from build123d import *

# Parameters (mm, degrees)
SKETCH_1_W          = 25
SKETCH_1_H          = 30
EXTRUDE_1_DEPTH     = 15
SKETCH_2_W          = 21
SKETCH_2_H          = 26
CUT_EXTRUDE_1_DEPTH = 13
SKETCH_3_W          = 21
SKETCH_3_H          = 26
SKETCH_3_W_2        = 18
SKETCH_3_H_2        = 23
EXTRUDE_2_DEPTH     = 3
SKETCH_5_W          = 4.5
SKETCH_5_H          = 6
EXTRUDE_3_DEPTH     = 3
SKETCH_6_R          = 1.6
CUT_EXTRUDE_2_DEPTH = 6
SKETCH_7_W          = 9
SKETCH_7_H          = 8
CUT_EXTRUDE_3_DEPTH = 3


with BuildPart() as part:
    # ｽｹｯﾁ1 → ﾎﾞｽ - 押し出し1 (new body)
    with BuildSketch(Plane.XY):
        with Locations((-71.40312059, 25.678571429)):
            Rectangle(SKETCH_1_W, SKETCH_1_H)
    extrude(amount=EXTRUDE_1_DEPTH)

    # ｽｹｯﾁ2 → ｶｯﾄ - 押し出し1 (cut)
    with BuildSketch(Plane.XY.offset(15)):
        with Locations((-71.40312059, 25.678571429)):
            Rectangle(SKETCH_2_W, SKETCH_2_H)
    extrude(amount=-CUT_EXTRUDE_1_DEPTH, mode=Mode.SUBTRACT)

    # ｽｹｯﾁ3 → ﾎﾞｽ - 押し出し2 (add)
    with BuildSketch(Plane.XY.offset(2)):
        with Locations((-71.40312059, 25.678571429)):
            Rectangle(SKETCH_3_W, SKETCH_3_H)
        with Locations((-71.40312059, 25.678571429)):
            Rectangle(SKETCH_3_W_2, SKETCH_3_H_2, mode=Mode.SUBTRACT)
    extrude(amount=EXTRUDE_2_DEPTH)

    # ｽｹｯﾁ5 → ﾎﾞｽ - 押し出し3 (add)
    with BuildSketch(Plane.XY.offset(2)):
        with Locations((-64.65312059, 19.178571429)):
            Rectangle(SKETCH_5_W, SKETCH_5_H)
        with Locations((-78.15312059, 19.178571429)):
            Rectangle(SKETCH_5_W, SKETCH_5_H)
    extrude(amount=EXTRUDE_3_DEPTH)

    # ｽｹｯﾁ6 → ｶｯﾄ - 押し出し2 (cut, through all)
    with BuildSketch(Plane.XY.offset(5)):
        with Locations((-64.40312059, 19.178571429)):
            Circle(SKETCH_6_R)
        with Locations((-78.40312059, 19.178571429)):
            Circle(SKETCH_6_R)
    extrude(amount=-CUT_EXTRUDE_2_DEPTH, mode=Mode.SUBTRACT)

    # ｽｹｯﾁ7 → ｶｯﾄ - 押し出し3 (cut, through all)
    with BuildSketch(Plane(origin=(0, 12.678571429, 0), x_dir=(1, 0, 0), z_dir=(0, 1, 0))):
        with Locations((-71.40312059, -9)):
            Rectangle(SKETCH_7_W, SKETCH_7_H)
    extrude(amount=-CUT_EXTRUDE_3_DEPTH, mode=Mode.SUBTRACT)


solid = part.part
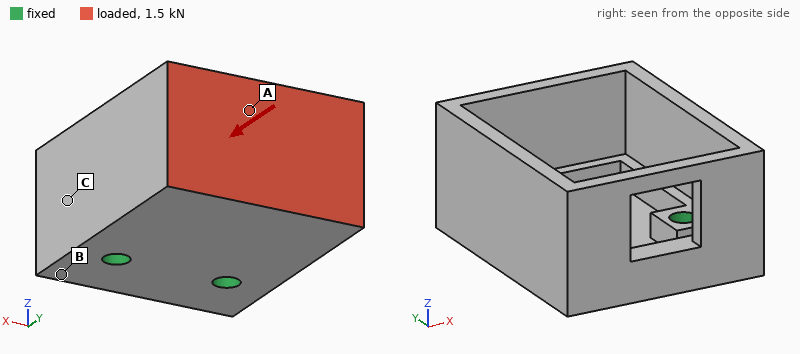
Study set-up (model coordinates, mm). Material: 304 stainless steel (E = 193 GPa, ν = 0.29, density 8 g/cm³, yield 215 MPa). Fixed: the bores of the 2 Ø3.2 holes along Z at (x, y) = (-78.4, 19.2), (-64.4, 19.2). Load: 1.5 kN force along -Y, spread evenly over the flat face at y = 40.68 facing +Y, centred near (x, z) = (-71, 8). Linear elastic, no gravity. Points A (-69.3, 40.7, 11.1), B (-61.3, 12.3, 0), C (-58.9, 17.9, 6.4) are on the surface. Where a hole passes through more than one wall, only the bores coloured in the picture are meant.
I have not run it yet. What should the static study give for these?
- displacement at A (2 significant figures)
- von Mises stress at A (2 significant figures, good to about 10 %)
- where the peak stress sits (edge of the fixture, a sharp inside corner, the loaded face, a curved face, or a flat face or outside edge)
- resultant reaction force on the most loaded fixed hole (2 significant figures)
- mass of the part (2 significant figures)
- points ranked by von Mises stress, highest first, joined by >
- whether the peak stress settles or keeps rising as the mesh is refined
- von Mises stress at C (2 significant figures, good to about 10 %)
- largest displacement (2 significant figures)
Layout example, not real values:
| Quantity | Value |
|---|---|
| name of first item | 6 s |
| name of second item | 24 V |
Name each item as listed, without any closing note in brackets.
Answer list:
| Quantity | Value |
|---|---|
| displacement at A | 38 µm |
| von Mises stress at A | 76 MPa |
| where the peak stress sits | edge of the fixture |
| resultant reaction force on the most loaded fixed hole | 750 N |
| mass of the part | 36 g |
| points ranked by von Mises stress, highest first, joined by > | A > C > B |
| whether the peak stress settles or keeps rising as the mesh is refined | keeps rising |
| von Mises stress at C | 36 MPa |
| largest displacement | 49 µm |
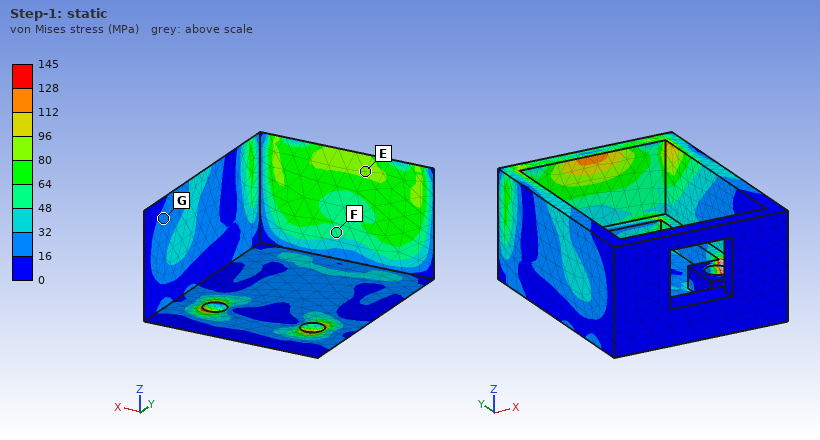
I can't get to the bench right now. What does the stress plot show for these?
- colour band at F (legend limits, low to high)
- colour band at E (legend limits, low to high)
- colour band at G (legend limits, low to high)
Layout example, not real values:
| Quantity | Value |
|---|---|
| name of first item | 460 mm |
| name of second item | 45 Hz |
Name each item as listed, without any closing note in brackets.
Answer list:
| Quantity | Value |
|---|---|
| colour band at F | 48 to 64 MPa |
| colour band at E | 80 to 96 MPa |
| colour band at G | 16 to 32 MPa |
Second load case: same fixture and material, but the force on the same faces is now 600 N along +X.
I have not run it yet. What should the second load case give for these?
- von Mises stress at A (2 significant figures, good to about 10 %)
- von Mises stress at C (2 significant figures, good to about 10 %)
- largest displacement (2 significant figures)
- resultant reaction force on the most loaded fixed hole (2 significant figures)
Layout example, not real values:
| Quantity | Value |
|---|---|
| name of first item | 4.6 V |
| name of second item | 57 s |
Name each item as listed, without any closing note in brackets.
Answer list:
| Quantity | Value |
|---|---|
| von Mises stress at A | 18 MPa |
| von Mises stress at C | 14 MPa |
| largest displacement | 29 µm |
| resultant reaction force on the most loaded fixed hole | 810 N |
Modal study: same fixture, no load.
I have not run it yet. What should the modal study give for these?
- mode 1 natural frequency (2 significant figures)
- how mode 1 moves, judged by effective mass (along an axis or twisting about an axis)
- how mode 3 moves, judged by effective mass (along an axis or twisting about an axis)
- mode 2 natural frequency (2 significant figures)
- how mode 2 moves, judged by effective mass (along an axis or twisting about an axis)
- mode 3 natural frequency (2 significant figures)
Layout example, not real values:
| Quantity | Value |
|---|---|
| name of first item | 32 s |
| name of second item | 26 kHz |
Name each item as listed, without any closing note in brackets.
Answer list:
| Quantity | Value |
|---|---|
| mode 1 natural frequency | 6100 Hz |
| how mode 1 moves, judged by effective mass | along Z |
| how mode 3 moves, judged by effective mass | along X |
| mode 2 natural frequency | 7100 Hz |
| how mode 2 moves, judged by effective mass | along X |
| mode 3 natural frequency | 15 kHz |
